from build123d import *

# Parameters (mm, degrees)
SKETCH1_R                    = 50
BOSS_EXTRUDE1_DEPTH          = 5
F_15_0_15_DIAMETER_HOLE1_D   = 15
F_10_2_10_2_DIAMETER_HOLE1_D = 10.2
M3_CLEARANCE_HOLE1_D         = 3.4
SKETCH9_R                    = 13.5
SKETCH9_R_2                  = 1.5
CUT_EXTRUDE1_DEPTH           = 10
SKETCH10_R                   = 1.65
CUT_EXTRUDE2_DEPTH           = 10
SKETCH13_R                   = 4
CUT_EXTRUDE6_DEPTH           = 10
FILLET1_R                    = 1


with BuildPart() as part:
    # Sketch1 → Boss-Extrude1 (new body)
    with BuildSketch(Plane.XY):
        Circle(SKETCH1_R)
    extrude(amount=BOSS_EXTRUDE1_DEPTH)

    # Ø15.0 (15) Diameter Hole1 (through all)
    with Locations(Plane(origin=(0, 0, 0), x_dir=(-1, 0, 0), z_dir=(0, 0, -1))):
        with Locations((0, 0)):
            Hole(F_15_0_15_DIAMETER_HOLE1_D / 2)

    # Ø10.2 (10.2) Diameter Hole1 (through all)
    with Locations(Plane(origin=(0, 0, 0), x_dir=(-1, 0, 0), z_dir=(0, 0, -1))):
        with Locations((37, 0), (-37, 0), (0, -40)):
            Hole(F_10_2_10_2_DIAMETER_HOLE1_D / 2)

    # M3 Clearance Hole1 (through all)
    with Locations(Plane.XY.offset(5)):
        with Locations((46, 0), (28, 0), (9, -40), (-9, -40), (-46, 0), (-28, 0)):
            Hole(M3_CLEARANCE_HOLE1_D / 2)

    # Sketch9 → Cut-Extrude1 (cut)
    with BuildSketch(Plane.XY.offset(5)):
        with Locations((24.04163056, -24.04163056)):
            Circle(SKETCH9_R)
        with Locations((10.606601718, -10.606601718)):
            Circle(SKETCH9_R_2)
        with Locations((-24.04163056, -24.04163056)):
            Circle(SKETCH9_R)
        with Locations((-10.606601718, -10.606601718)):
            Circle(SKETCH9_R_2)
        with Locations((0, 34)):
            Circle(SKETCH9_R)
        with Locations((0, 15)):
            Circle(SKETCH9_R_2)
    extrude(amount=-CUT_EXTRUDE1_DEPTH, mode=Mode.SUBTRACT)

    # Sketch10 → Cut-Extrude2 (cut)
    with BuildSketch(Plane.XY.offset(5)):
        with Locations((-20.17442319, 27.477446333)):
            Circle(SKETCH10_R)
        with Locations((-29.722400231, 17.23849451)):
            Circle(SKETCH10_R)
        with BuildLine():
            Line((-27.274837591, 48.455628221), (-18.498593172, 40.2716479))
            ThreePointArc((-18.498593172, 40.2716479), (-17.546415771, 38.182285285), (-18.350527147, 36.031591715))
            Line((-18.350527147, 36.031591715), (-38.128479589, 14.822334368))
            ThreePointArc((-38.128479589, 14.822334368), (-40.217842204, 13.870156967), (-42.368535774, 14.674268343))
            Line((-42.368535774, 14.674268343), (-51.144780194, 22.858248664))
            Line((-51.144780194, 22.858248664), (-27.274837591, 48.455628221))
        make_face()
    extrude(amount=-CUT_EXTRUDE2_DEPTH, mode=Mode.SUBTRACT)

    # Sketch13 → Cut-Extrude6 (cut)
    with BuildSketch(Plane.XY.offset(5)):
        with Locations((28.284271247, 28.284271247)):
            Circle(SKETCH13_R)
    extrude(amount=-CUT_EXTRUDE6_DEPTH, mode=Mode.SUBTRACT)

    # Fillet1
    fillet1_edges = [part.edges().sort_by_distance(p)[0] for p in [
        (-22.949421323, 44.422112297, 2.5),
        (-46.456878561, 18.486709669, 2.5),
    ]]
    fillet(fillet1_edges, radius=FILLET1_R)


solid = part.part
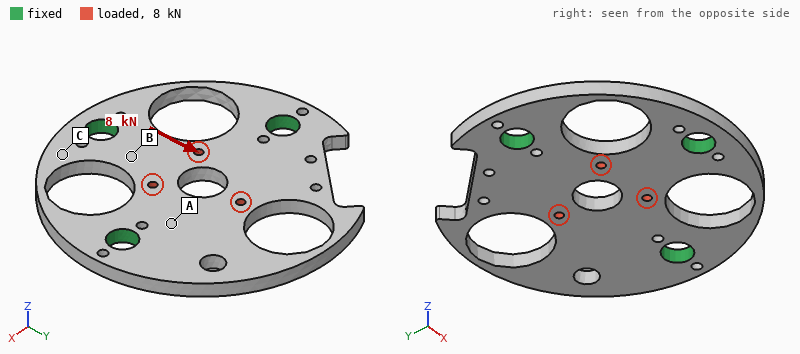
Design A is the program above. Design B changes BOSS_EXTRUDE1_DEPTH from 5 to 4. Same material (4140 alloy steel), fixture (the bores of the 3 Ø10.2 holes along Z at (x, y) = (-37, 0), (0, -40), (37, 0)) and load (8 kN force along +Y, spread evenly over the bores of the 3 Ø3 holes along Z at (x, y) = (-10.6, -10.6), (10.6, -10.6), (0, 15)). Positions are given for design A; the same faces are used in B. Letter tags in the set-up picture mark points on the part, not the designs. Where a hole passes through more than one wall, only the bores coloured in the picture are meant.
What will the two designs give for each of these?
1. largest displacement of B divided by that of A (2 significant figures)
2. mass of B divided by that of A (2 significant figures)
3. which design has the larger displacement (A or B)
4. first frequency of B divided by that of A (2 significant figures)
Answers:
1.2
0.80
B
0.81
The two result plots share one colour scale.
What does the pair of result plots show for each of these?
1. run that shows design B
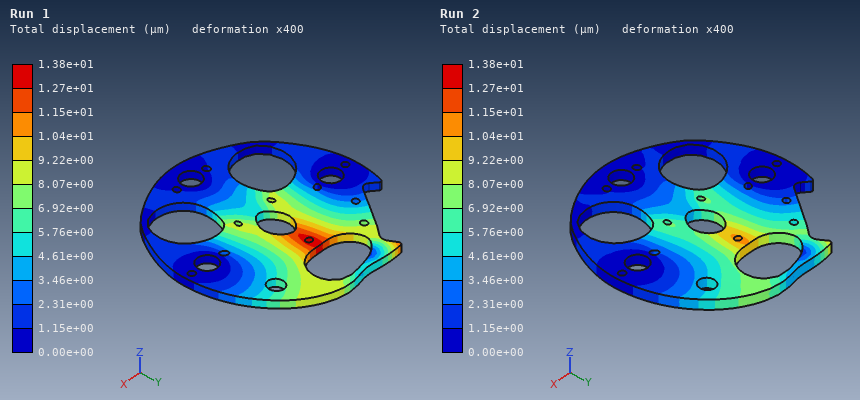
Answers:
Run 1
